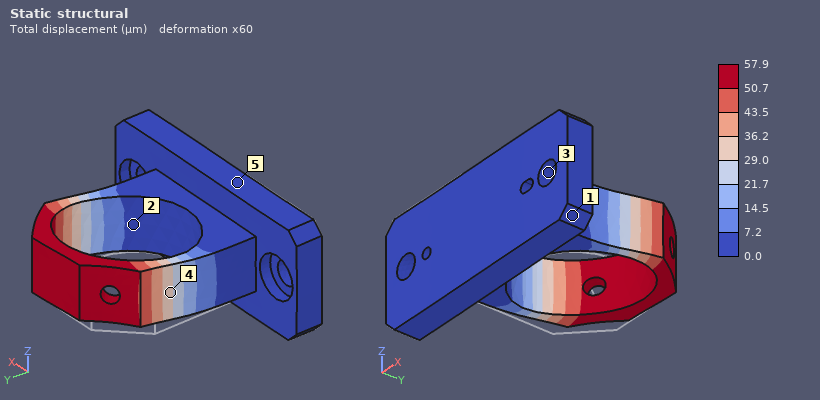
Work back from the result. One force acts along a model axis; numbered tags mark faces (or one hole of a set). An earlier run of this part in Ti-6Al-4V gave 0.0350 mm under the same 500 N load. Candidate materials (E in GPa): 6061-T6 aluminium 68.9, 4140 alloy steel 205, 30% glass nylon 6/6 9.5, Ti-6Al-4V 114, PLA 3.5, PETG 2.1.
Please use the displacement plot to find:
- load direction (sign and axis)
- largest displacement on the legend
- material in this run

+X
57.9 µm
6061-T6 aluminium
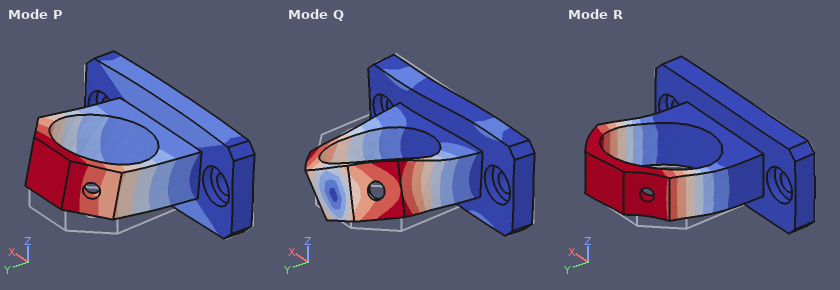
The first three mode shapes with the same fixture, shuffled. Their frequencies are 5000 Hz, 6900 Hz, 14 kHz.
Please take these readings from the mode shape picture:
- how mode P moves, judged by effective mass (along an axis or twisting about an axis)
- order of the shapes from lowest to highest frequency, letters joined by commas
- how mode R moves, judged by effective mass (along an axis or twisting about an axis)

along Z
P, R, Q
along X
